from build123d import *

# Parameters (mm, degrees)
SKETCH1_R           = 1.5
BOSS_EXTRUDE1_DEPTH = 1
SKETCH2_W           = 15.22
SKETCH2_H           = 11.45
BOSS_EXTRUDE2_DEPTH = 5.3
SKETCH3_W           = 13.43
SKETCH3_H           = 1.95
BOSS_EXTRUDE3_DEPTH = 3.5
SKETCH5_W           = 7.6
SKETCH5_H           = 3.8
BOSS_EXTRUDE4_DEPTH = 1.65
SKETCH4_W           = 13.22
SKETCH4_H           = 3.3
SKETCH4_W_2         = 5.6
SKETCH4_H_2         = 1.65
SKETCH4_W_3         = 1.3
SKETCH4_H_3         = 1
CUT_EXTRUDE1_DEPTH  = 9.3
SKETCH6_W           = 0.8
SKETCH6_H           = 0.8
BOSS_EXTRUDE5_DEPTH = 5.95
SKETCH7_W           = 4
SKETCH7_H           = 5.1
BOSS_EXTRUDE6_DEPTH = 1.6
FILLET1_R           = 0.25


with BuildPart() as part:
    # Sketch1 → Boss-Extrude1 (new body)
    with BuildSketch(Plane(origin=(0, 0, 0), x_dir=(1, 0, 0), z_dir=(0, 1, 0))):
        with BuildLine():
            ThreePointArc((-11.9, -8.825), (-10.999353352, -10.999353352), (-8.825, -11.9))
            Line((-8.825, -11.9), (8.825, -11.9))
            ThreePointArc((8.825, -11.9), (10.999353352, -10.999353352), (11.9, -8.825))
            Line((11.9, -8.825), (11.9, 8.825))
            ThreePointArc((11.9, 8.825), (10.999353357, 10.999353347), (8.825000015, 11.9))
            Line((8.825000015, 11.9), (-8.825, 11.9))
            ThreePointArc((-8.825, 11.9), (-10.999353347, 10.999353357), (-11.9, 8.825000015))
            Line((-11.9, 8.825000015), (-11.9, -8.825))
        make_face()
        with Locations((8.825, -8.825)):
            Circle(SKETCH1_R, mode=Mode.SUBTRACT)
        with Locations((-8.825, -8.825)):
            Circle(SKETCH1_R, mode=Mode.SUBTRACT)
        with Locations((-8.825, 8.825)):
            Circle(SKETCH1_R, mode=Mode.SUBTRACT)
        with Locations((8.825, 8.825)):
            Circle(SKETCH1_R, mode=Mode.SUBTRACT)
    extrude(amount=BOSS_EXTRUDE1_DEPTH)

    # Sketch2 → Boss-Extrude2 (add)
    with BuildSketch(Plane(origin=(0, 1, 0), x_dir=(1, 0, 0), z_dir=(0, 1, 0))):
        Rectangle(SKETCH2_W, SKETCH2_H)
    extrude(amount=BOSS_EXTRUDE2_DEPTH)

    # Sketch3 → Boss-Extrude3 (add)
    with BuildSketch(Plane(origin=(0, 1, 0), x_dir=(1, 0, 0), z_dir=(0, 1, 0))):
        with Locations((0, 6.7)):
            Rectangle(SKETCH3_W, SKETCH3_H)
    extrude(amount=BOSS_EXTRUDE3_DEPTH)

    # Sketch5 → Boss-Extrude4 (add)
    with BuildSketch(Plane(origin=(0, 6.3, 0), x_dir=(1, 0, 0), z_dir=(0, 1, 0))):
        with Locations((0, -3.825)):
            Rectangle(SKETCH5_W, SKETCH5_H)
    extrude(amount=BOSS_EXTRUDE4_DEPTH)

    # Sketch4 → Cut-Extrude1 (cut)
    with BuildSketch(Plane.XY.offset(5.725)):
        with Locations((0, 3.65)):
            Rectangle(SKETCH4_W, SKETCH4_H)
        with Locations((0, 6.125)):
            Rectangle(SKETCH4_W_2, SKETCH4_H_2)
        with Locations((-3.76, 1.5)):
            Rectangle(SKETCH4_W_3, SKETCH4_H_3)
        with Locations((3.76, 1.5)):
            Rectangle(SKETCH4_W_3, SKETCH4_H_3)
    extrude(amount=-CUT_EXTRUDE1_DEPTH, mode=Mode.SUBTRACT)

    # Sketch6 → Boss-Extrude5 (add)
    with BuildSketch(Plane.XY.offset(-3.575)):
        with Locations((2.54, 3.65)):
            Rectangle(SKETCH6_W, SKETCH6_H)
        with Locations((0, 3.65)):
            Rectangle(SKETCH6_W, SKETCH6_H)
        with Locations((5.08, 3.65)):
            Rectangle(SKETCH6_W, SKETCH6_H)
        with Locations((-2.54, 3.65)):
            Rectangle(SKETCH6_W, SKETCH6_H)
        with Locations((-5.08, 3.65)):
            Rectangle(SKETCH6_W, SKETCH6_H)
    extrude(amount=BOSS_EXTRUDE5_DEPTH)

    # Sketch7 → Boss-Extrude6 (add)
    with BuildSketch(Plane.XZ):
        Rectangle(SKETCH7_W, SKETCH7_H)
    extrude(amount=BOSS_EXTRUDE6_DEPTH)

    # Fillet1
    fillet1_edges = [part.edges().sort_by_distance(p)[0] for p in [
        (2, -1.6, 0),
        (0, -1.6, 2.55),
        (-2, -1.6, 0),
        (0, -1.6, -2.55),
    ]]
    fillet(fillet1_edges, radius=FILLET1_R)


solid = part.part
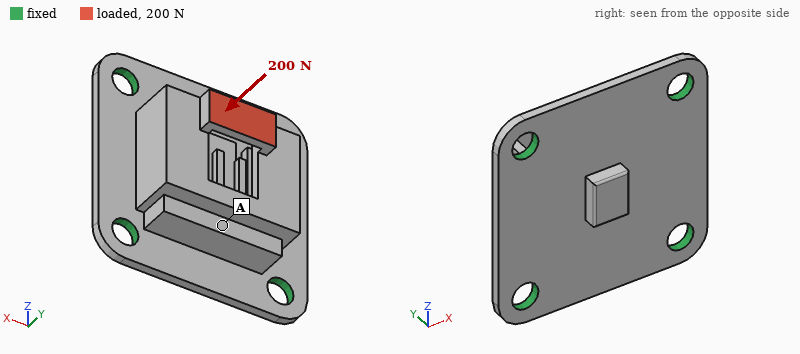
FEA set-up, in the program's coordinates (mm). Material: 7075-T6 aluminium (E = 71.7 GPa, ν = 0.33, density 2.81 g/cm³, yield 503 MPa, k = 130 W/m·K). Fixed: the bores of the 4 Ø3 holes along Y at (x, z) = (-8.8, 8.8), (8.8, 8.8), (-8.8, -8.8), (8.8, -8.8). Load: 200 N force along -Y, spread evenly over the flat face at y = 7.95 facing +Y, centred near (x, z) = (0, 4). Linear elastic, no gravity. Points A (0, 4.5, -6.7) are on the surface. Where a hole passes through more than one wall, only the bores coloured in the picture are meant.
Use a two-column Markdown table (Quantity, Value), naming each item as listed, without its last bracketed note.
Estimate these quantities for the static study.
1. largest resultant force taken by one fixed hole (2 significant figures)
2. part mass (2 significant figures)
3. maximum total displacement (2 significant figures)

| Quantity | Value |
|---|---|
| largest resultant force taken by one fixed hole | 89 N |
| part mass | 3.2 g |
| maximum total displacement | 70 µm |
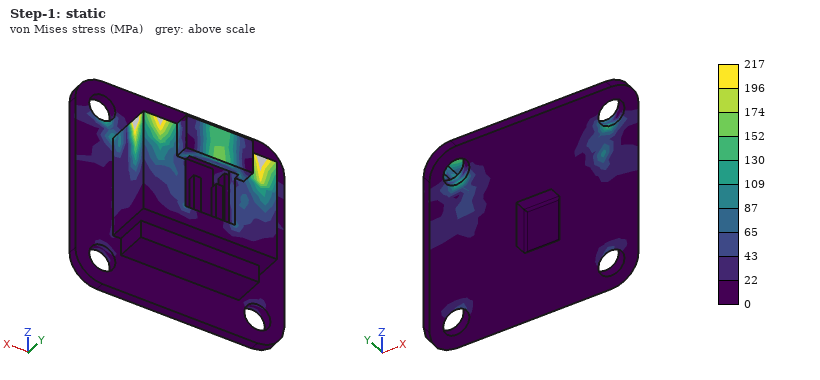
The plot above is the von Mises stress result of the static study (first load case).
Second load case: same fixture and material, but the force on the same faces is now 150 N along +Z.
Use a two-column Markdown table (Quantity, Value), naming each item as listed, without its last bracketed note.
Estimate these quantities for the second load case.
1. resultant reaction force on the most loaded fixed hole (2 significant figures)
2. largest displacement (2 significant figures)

| Quantity | Value |
|---|---|
| resultant reaction force on the most loaded fixed hole | 58 N |
| largest displacement | 39 µm |
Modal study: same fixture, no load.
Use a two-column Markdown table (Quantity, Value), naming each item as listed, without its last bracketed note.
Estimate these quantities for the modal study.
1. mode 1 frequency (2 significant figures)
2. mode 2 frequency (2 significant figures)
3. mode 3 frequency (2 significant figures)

| Quantity | Value |
|---|---|
| mode 1 frequency | 17 kHz |
| mode 2 frequency | 18 kHz |
| mode 3 frequency | 18 kHz |
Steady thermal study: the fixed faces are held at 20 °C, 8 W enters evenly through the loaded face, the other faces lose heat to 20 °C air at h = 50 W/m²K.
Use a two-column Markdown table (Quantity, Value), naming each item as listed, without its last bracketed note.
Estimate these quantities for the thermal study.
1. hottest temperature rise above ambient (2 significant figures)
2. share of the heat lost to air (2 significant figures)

| Quantity | Value |
|---|---|
| hottest temperature rise above ambient | 55 K |
| share of the heat lost to air | 9.6 % |
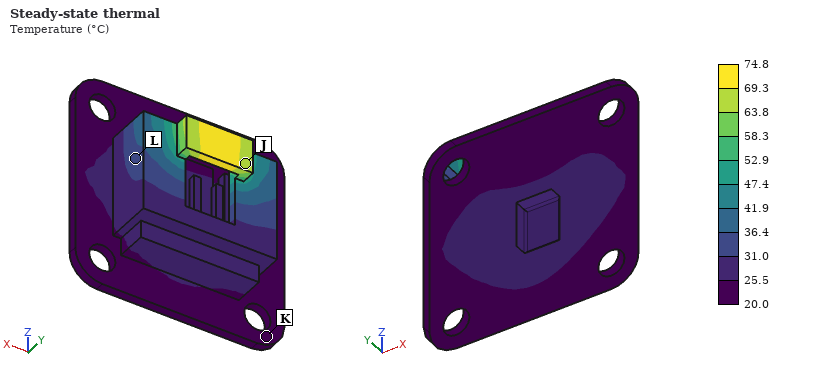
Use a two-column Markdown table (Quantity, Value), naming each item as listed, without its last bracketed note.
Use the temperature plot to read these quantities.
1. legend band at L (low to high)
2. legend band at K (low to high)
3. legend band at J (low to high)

| Quantity | Value |
|---|---|
| legend band at L | 31.0 to 36.4 °C |
| legend band at K | 20.0 to 25.5 °C |
| legend band at J | 63.8 to 69.3 °C |
